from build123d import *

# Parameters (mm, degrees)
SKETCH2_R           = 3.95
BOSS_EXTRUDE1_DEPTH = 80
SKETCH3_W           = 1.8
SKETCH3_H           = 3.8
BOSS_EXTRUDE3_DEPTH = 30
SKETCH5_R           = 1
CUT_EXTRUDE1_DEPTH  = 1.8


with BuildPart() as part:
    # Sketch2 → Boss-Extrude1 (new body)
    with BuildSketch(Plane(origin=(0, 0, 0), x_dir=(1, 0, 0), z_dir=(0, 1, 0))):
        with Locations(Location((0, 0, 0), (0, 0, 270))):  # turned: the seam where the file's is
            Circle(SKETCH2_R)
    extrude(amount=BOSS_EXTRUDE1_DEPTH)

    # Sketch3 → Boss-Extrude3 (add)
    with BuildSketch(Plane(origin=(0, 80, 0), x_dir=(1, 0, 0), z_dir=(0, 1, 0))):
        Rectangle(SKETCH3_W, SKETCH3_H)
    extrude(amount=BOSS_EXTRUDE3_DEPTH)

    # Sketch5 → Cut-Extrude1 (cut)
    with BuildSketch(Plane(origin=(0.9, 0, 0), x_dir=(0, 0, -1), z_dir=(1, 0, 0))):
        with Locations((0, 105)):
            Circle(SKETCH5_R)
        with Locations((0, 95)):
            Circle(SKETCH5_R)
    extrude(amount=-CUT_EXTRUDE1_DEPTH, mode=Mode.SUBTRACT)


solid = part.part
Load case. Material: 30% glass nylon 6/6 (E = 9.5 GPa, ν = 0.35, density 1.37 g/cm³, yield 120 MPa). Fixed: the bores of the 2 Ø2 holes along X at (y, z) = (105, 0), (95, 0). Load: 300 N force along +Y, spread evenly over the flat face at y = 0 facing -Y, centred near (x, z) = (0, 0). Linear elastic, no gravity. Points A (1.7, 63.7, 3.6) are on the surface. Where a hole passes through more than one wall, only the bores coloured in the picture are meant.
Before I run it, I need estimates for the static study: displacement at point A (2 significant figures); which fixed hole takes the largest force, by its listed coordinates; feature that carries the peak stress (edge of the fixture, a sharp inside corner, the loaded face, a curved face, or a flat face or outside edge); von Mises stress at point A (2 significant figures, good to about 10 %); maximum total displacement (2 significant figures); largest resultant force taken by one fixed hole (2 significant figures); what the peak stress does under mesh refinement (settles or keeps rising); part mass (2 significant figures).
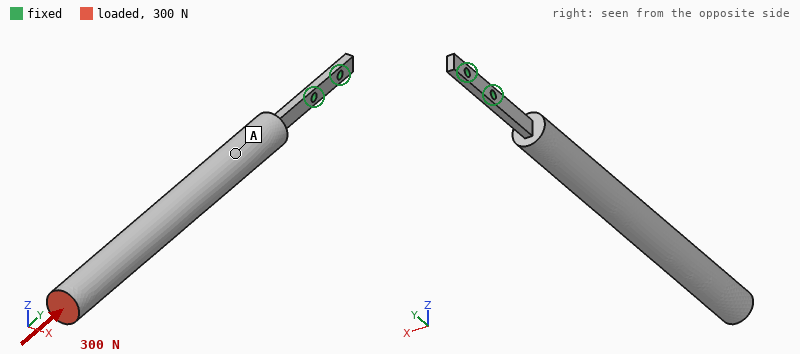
0.082 mm
(95, 0)
edge of the fixture
6.1 MPa
0.12 mm
300 N
keeps rising
5.6 g
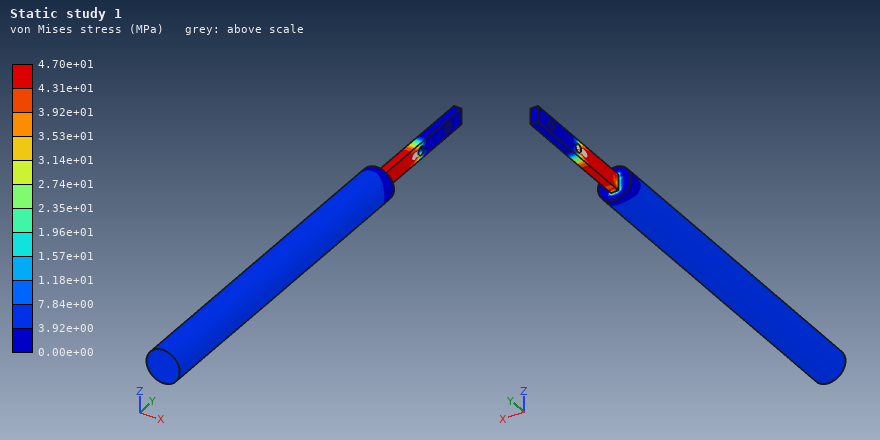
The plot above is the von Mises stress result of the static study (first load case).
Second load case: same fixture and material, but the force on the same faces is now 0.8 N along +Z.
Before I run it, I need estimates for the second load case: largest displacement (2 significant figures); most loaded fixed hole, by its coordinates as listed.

1.3 mm
(95, 0)
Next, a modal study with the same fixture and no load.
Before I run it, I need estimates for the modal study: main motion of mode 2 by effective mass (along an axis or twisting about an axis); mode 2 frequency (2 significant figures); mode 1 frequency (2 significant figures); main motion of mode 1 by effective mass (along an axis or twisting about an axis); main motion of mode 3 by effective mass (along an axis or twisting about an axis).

along Z
90 Hz
45 Hz
along X
twisting about Y
